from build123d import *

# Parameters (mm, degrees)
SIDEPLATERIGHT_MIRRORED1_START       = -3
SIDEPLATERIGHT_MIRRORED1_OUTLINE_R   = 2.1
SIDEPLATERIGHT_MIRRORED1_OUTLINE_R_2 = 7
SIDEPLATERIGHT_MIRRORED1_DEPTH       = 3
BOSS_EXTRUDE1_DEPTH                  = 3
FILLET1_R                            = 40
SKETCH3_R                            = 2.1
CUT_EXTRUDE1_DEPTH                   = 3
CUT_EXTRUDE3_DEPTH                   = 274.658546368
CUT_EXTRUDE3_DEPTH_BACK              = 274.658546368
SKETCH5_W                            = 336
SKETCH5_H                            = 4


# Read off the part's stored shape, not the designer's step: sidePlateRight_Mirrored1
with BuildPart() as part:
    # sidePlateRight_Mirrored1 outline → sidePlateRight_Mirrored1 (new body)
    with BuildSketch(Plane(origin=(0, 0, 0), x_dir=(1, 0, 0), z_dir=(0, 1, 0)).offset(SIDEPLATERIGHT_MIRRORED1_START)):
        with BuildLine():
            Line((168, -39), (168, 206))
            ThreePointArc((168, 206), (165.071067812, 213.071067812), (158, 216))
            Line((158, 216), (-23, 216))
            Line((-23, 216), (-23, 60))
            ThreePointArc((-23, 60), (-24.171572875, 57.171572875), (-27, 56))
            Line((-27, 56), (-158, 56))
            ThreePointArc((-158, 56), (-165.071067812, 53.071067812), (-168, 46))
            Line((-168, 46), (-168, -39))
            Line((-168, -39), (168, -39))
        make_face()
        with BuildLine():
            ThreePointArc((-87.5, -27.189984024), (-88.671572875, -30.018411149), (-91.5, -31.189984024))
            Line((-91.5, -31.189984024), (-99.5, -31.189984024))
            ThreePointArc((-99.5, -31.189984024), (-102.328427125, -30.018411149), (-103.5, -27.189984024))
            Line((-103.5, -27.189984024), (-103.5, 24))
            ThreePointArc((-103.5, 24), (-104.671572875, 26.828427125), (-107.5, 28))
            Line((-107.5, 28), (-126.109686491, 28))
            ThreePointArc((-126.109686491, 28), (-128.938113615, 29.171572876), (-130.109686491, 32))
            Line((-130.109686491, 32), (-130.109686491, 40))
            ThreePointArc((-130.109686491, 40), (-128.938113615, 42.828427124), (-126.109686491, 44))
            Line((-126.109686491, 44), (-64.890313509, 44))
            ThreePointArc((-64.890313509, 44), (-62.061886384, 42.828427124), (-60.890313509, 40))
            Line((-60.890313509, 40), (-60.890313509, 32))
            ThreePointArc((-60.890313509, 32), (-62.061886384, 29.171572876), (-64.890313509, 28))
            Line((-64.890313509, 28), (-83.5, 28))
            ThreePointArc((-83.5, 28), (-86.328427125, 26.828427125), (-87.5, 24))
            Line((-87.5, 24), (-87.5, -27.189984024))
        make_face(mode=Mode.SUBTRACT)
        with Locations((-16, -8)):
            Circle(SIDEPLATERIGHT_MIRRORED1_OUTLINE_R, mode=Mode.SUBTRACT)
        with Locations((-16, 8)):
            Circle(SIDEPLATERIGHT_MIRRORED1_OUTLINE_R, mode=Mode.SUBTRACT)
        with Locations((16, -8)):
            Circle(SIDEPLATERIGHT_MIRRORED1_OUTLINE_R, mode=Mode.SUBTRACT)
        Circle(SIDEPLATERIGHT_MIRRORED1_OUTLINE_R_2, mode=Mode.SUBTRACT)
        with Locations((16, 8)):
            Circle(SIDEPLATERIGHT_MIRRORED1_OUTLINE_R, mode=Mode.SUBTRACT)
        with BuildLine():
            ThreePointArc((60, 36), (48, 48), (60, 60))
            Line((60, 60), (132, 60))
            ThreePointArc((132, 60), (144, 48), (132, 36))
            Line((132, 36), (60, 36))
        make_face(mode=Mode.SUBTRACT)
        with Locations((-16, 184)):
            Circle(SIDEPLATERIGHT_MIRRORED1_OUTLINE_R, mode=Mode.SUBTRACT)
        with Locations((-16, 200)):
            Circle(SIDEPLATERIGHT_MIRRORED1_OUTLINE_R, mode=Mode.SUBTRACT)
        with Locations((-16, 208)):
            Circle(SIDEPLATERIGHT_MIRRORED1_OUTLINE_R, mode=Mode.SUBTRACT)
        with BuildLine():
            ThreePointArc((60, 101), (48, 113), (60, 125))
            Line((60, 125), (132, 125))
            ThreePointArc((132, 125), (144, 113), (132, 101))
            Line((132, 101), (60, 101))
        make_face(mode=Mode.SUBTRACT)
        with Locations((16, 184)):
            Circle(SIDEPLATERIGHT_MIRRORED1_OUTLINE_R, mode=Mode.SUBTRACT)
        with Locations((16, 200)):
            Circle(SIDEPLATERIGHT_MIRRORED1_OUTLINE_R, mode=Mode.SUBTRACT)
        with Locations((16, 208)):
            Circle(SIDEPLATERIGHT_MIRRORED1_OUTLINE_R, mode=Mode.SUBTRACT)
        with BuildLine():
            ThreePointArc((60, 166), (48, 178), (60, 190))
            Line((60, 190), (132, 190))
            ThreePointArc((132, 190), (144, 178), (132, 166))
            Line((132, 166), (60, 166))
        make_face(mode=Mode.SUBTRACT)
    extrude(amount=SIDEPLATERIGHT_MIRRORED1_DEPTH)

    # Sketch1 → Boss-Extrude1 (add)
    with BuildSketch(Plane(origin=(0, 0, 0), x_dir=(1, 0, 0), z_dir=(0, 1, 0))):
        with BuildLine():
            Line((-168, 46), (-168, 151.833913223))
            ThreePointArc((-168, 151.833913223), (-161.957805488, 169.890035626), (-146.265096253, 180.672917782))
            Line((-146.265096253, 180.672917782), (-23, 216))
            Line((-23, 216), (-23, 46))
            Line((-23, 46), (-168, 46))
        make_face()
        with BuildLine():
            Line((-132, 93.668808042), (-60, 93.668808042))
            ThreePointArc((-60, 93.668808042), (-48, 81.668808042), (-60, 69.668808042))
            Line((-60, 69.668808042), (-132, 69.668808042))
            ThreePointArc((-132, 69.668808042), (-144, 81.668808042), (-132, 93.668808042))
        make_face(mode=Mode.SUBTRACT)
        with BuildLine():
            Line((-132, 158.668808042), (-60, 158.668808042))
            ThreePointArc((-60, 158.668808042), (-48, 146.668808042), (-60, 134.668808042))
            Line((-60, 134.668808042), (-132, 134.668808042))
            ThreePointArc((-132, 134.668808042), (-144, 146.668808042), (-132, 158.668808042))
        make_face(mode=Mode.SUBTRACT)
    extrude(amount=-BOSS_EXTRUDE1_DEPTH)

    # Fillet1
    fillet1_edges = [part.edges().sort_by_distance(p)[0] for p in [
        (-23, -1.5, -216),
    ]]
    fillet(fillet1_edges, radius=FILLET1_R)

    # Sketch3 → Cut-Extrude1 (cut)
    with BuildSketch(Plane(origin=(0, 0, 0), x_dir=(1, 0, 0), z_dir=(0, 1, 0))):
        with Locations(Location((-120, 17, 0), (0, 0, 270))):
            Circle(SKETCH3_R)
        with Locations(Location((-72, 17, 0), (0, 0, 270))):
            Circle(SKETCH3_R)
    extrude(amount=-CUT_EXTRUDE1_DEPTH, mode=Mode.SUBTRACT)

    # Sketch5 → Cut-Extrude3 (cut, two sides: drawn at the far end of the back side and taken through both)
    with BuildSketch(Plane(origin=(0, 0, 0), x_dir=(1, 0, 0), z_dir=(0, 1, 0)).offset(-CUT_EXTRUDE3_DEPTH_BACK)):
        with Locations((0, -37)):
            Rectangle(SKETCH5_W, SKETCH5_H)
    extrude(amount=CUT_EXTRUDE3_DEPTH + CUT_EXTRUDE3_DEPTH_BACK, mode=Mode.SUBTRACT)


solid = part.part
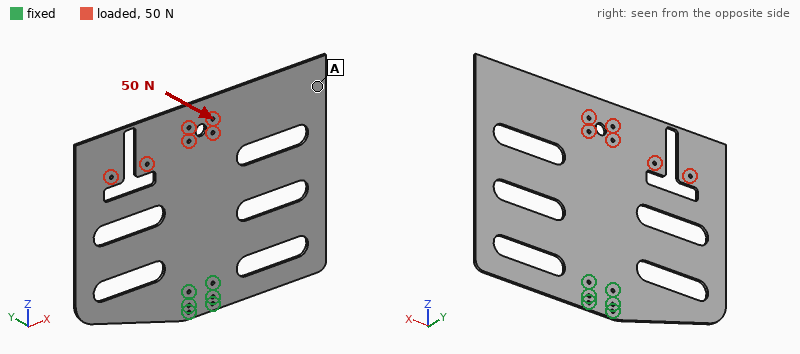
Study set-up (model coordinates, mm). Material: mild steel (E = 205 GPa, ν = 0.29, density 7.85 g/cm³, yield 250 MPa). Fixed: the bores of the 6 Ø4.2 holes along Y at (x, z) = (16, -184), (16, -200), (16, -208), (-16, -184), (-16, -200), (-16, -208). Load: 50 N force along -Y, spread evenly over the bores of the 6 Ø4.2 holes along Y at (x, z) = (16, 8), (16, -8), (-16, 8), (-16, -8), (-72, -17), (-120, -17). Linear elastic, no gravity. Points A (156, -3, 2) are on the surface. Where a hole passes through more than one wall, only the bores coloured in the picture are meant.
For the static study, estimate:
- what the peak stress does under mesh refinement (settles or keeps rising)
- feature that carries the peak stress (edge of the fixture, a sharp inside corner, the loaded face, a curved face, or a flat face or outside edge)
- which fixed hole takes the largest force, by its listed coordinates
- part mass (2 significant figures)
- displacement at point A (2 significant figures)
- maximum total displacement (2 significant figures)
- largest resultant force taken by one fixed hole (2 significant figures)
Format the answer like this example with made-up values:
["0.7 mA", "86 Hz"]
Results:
["keeps rising", "edge of the fixture", "(-16, -184)", "1.6 kg", "1.2 mm", "2.2 mm", "200 N"]
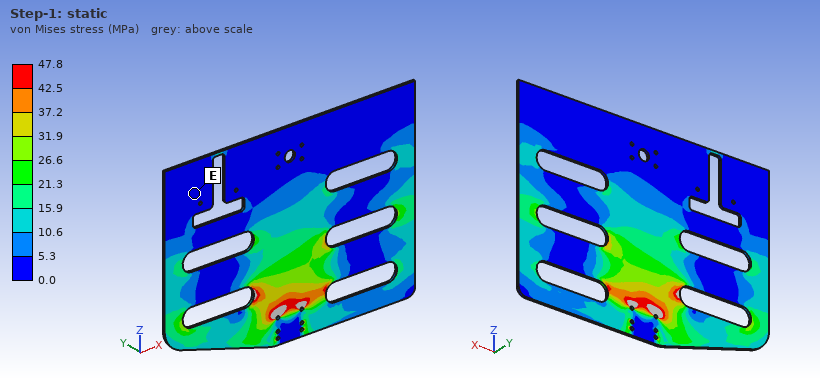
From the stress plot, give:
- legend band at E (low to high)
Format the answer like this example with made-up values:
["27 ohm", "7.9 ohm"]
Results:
["0.0 to 5.3 MPa"]
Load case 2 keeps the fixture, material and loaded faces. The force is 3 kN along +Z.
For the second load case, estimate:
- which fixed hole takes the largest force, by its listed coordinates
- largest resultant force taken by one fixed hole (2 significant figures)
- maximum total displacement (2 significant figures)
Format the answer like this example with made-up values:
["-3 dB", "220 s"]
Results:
["(-16, -184)", "2.2 kN", "55 µm"]
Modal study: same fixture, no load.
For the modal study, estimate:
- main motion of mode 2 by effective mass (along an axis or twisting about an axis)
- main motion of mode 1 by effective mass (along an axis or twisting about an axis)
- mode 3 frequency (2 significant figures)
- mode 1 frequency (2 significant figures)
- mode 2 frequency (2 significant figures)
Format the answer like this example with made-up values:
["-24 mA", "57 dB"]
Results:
["twisting about Z", "along Y", "110 Hz", "35 Hz", "50 Hz"]
